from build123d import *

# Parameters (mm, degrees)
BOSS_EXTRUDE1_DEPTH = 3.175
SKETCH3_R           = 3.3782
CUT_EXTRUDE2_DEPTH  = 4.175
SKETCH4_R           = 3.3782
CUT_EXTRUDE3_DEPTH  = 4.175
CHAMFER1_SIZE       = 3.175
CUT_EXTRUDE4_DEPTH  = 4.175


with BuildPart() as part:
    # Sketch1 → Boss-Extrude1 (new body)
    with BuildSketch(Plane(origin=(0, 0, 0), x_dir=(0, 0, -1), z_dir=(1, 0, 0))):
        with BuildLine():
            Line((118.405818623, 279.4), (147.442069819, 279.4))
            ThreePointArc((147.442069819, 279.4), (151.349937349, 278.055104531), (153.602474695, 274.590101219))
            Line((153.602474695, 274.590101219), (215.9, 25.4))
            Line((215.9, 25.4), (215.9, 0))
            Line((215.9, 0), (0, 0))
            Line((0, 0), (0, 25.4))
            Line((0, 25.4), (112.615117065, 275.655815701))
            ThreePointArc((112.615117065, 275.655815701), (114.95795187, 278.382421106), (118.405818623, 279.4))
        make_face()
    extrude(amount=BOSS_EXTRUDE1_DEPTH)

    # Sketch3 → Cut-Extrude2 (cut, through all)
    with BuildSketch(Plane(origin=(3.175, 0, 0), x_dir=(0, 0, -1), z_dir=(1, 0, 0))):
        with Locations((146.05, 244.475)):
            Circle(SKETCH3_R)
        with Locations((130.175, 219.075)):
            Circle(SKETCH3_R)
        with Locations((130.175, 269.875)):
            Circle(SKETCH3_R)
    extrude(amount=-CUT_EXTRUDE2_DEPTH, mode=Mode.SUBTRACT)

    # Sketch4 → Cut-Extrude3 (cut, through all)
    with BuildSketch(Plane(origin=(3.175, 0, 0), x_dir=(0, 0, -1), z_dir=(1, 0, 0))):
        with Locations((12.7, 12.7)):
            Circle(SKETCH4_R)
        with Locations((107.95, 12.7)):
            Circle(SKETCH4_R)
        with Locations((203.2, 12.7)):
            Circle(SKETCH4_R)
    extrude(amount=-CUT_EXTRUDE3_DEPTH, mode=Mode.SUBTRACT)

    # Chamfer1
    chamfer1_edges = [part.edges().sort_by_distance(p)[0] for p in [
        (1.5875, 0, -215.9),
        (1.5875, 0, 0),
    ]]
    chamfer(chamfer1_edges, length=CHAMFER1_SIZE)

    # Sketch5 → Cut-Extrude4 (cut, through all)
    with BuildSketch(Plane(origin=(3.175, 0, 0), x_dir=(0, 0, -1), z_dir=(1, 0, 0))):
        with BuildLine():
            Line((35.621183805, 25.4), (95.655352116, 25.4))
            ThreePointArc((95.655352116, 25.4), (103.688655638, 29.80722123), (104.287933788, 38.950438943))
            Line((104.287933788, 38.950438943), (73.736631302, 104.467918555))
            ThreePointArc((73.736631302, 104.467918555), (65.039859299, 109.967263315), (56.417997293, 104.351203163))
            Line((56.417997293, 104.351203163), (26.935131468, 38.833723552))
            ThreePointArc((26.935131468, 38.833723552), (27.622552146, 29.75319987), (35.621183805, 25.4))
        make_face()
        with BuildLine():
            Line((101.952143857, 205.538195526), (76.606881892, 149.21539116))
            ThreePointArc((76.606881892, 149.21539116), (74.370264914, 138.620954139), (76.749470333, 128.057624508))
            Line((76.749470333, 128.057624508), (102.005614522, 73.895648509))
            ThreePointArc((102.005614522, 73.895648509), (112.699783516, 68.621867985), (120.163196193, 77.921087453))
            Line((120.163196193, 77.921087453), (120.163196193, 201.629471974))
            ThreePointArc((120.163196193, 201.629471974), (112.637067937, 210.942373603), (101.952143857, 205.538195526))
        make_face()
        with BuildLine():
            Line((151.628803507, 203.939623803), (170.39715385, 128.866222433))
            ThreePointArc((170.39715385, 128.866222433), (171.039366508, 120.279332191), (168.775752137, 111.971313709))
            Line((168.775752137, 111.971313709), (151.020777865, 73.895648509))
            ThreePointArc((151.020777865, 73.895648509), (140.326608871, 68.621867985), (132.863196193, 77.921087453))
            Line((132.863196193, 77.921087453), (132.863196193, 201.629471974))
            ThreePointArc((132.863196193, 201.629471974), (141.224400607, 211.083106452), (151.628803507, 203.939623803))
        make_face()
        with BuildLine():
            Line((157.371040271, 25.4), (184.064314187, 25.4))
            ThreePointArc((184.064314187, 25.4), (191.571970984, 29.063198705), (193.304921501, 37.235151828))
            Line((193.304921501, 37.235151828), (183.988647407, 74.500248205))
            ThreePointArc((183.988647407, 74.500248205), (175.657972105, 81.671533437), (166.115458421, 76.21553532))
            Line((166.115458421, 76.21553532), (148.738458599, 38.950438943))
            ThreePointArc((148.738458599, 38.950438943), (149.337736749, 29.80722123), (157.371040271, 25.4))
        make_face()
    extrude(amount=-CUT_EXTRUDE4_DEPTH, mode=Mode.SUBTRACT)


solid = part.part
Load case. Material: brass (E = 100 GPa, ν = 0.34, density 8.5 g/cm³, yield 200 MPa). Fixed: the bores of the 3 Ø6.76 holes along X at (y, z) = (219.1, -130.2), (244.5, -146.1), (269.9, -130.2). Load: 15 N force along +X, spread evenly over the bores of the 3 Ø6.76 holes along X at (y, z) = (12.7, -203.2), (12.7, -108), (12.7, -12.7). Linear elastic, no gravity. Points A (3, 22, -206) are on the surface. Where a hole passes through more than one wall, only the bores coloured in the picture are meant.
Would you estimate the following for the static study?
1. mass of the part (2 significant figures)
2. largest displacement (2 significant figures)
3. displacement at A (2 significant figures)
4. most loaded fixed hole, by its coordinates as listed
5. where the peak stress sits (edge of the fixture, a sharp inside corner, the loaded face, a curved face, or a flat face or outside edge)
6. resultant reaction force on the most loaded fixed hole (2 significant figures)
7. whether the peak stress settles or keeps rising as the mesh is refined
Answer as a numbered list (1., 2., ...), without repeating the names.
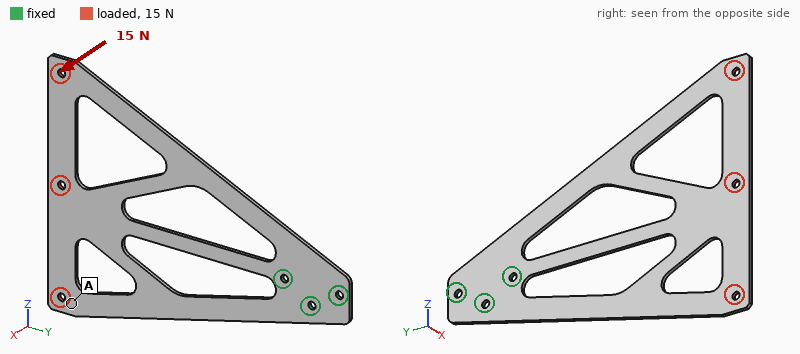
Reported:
1. 620 g
2. 4.0 mm
3. 2.9 mm
4. (219.1, -130.2)
5. edge of the fixture
6. 69 N
7. keeps rising
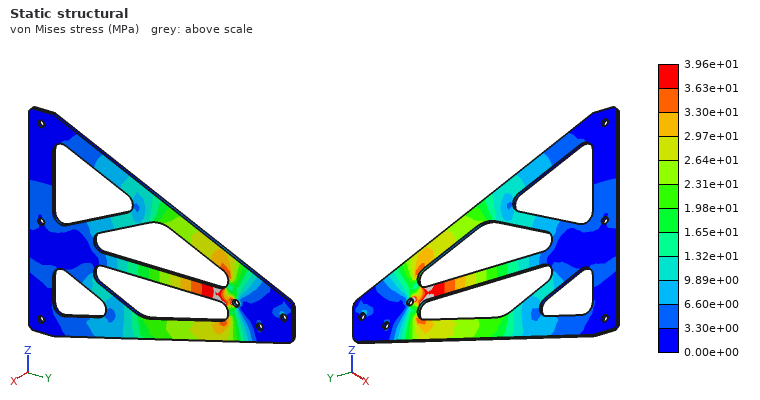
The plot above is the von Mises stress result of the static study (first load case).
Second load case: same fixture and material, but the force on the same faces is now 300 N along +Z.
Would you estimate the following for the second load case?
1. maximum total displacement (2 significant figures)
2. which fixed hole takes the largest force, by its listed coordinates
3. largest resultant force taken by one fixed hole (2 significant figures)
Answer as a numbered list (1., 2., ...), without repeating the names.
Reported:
1. 0.49 mm
2. (219.1, -130.2)
3. 1.5 kN
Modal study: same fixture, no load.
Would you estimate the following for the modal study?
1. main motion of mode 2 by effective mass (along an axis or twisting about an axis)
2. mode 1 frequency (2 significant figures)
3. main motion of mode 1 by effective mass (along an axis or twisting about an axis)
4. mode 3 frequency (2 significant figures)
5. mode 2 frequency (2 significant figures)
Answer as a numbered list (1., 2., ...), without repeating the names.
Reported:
1. twisting about Y
2. 22 Hz
3. along X
4. 160 Hz
5. 51 Hz
